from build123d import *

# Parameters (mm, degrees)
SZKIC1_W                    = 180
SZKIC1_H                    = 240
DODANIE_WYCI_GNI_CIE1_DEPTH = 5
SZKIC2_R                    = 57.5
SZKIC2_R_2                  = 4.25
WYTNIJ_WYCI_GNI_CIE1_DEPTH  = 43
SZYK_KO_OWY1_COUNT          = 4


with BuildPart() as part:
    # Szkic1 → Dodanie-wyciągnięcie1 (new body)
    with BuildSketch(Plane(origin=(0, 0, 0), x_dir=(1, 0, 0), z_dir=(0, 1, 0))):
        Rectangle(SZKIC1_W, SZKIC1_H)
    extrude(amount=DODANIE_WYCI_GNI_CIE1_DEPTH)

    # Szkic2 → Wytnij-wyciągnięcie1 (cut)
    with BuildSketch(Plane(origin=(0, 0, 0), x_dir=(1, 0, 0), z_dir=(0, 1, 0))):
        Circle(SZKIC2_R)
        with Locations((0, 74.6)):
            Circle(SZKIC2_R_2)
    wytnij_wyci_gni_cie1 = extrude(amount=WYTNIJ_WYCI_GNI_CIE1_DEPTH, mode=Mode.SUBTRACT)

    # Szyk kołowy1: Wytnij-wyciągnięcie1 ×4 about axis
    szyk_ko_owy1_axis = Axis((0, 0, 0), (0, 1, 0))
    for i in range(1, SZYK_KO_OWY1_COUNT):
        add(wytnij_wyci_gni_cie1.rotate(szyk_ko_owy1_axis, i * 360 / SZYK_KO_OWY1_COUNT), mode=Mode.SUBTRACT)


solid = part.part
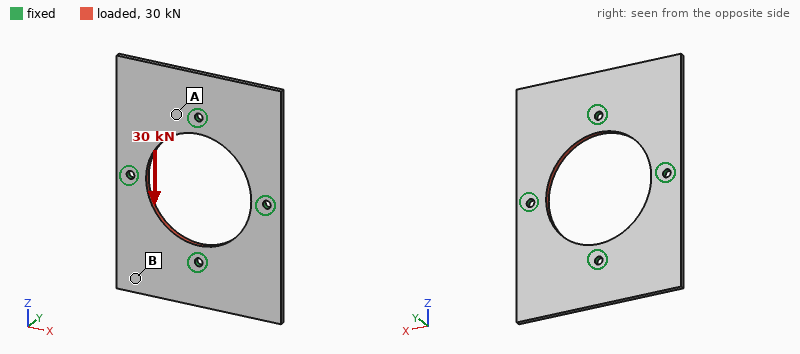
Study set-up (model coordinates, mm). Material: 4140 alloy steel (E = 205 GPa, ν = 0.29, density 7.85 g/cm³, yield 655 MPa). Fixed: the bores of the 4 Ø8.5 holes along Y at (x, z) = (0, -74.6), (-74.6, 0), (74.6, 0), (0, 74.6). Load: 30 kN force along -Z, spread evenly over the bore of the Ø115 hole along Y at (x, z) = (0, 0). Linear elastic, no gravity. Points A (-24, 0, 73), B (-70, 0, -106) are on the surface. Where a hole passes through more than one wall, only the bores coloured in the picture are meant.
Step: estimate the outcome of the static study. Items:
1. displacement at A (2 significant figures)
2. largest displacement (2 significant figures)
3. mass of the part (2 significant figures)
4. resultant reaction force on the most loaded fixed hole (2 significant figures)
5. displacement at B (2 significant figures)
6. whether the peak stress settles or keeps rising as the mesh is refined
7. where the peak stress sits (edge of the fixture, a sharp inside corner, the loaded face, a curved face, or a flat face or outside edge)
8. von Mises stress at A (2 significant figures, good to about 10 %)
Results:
4.7 µm
8.5 µm
1.3 kg
8.4 kN
5.8 µm
keeps rising
edge of the fixture
17 MPa
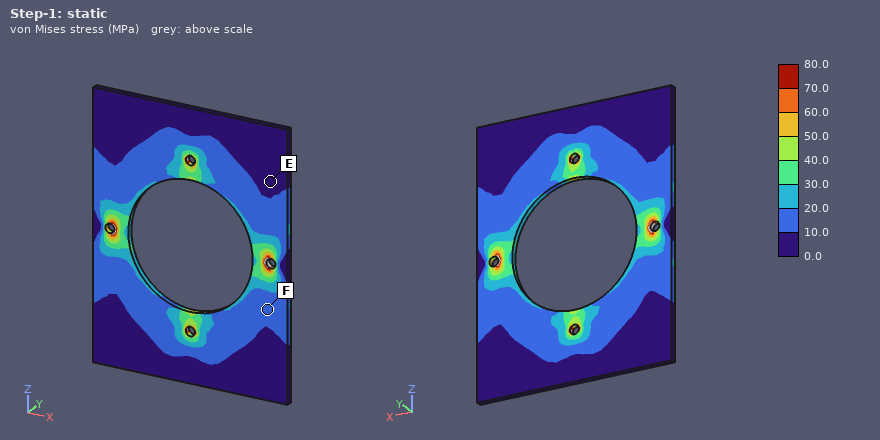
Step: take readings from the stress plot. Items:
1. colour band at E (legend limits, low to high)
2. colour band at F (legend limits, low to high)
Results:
0.0 to 10.0 MPa
10.0 to 20.0 MPa
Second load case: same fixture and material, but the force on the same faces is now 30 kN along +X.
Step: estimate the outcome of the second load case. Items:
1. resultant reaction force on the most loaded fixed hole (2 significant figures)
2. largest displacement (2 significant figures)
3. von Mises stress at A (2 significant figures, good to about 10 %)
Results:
8.8 kN
9.3 µm
20 MPa
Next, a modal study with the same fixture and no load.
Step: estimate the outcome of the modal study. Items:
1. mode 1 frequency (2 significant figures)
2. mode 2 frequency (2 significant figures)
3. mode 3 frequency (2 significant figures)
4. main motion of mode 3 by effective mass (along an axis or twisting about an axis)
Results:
630 Hz
630 Hz
710 Hz
along Y
